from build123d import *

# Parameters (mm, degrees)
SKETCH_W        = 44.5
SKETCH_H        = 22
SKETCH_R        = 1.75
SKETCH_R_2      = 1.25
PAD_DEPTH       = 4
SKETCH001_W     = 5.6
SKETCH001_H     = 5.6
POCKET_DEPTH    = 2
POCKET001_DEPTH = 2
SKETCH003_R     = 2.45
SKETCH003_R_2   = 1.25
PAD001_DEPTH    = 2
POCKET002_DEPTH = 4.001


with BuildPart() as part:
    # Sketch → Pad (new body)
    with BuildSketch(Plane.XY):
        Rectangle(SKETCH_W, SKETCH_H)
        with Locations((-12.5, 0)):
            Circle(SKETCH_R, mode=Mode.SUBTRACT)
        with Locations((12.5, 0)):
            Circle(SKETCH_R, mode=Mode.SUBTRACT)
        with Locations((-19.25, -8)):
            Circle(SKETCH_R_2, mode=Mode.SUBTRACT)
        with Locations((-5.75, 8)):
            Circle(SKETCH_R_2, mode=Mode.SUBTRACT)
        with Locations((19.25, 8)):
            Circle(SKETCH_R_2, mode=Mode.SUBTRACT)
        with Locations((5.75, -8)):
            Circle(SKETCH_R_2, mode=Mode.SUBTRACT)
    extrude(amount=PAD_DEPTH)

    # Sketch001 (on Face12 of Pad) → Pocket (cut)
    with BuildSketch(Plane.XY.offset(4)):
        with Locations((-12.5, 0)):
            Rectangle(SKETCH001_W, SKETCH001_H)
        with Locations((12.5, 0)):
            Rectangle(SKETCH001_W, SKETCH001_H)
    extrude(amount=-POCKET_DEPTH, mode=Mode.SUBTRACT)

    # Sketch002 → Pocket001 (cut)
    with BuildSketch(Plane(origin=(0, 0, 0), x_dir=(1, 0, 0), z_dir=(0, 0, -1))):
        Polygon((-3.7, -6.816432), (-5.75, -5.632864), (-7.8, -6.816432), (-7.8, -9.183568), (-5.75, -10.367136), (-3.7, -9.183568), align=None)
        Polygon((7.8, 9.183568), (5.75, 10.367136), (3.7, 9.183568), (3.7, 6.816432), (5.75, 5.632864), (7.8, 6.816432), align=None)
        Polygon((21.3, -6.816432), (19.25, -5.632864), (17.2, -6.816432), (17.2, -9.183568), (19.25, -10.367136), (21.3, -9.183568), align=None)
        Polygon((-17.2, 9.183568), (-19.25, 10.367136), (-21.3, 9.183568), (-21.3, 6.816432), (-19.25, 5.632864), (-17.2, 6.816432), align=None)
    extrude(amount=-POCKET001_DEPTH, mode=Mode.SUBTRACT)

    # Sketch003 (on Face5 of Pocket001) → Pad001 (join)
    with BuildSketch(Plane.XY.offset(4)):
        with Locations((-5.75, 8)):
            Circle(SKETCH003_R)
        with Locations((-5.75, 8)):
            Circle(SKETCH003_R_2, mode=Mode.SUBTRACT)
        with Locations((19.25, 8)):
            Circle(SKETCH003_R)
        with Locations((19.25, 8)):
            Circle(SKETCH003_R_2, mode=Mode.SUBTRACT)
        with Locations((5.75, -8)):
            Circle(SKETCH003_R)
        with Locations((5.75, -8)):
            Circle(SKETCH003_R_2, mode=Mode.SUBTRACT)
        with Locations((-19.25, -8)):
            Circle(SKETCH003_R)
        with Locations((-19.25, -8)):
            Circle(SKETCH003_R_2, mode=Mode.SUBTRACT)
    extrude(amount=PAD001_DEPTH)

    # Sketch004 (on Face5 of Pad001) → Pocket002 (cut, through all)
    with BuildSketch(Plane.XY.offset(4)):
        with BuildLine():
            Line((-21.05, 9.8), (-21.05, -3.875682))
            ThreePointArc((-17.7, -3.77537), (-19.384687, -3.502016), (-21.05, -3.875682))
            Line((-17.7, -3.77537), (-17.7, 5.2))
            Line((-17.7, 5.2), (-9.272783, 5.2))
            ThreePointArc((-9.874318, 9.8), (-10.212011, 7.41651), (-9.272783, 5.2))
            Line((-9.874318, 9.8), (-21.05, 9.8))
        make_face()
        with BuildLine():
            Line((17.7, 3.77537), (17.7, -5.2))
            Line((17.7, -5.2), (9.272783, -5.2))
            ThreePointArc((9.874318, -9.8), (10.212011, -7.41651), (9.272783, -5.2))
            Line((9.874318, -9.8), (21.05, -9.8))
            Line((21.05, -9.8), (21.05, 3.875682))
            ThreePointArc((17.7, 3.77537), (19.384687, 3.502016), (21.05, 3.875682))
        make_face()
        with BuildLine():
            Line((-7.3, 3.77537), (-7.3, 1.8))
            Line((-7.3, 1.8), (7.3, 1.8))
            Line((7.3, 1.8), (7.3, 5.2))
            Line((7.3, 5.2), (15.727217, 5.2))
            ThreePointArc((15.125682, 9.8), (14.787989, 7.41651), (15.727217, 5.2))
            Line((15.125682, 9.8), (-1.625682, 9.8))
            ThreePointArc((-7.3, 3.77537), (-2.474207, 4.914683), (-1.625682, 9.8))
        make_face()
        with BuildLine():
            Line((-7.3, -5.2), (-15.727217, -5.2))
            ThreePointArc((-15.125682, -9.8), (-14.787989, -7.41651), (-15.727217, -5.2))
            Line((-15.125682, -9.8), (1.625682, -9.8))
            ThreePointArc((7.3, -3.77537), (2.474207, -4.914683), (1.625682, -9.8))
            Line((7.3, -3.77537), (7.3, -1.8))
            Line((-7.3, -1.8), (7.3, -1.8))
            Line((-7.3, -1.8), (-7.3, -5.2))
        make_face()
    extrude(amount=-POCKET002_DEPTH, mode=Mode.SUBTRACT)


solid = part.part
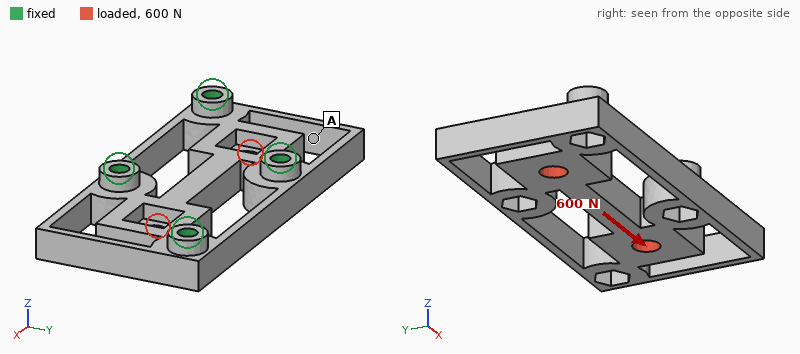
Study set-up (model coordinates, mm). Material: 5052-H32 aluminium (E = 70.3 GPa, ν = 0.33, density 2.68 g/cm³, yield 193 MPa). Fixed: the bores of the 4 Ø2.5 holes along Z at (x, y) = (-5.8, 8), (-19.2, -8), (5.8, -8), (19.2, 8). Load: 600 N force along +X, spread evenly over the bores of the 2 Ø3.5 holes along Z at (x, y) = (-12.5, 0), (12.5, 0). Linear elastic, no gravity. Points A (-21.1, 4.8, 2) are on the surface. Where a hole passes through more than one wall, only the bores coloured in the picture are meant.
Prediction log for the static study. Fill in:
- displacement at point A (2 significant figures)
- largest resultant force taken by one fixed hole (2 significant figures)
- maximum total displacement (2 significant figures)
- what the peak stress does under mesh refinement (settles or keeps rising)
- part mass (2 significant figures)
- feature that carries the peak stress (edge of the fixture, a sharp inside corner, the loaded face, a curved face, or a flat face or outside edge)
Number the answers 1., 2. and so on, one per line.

1. 2.3 µm
2. 150 N
3. 6.6 µm
4. keeps rising
5. 5.7 g
6. edge of the fixture
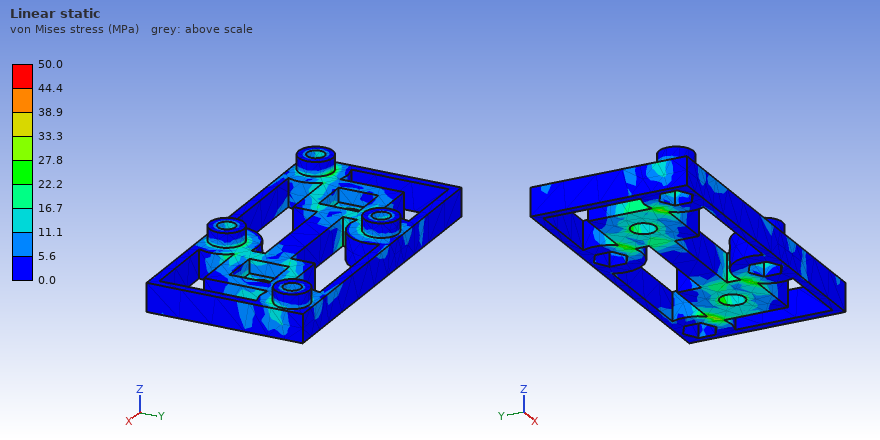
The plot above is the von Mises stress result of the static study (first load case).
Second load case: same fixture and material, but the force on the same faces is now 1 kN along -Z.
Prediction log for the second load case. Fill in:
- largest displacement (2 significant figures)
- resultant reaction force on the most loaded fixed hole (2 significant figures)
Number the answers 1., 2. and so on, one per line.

1. 21 µm
2. 340 N
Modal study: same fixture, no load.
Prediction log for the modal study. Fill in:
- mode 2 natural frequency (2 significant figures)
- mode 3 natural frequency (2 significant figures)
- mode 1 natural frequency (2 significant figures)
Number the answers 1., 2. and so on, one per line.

1. 13 kHz
2. 19 kHz
3. 13 kHz
